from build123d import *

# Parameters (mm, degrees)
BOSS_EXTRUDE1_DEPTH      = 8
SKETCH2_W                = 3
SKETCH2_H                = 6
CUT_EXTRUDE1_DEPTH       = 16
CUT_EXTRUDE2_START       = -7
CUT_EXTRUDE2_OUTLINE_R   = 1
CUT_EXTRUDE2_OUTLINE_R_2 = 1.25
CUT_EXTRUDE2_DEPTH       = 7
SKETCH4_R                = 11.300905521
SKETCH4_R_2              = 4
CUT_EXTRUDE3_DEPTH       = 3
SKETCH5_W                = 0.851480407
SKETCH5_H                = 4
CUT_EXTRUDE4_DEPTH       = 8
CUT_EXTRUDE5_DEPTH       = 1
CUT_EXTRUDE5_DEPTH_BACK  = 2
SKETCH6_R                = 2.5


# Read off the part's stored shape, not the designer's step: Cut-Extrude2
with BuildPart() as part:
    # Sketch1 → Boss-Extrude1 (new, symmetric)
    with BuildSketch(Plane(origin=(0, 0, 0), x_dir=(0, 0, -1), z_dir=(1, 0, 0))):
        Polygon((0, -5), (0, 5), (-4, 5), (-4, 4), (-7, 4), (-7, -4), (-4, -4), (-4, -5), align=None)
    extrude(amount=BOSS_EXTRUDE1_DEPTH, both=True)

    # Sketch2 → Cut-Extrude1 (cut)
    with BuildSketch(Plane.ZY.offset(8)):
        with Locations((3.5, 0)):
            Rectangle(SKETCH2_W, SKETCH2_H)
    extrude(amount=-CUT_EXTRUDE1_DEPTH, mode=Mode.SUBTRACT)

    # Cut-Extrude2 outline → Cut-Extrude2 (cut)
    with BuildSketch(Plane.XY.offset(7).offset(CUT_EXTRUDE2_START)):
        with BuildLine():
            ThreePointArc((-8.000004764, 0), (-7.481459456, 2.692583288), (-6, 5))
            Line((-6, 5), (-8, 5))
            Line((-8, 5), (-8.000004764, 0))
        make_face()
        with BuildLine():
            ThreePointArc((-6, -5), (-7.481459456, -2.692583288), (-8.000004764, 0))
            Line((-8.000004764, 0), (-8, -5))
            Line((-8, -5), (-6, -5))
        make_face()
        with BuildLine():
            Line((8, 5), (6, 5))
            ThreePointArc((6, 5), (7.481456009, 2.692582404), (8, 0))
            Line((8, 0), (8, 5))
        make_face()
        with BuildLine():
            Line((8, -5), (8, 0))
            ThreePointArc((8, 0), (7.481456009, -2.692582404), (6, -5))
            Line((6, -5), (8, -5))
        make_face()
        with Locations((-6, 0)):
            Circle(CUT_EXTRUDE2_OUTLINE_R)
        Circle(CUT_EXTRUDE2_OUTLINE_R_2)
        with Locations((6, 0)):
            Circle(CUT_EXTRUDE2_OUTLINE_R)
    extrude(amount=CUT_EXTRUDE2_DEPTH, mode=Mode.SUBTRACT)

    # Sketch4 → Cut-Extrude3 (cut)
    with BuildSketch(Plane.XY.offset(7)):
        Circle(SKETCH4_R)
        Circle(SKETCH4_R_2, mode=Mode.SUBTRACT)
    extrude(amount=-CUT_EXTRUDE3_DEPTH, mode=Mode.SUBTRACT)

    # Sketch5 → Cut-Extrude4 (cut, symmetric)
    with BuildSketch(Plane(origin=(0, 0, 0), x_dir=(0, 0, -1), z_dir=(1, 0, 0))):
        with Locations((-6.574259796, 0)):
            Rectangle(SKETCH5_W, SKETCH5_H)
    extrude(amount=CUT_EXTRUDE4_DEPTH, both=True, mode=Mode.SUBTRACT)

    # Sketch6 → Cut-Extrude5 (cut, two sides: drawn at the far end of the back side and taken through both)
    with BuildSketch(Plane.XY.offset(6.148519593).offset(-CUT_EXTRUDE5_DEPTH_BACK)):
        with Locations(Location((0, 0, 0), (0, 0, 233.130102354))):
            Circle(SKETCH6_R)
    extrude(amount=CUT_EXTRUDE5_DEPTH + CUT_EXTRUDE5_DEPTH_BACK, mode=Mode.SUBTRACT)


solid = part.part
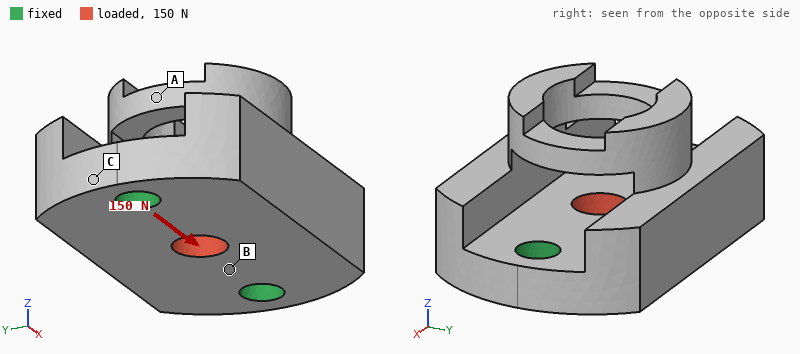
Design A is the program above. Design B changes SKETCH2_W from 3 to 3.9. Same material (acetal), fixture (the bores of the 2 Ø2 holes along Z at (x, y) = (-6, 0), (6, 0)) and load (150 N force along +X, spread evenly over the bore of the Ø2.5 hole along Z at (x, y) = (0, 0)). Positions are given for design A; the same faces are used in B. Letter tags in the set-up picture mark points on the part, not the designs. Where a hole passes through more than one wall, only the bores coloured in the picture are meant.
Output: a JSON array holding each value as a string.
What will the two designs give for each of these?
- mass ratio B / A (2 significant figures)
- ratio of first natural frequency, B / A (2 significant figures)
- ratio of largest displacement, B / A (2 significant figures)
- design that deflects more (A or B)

["0.89", "0.77", "1.3", "B"]
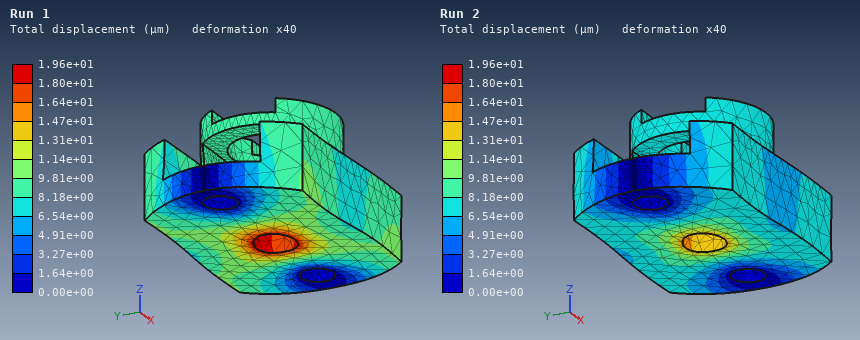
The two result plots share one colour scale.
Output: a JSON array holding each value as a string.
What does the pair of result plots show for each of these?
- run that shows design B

["Run 1"]
